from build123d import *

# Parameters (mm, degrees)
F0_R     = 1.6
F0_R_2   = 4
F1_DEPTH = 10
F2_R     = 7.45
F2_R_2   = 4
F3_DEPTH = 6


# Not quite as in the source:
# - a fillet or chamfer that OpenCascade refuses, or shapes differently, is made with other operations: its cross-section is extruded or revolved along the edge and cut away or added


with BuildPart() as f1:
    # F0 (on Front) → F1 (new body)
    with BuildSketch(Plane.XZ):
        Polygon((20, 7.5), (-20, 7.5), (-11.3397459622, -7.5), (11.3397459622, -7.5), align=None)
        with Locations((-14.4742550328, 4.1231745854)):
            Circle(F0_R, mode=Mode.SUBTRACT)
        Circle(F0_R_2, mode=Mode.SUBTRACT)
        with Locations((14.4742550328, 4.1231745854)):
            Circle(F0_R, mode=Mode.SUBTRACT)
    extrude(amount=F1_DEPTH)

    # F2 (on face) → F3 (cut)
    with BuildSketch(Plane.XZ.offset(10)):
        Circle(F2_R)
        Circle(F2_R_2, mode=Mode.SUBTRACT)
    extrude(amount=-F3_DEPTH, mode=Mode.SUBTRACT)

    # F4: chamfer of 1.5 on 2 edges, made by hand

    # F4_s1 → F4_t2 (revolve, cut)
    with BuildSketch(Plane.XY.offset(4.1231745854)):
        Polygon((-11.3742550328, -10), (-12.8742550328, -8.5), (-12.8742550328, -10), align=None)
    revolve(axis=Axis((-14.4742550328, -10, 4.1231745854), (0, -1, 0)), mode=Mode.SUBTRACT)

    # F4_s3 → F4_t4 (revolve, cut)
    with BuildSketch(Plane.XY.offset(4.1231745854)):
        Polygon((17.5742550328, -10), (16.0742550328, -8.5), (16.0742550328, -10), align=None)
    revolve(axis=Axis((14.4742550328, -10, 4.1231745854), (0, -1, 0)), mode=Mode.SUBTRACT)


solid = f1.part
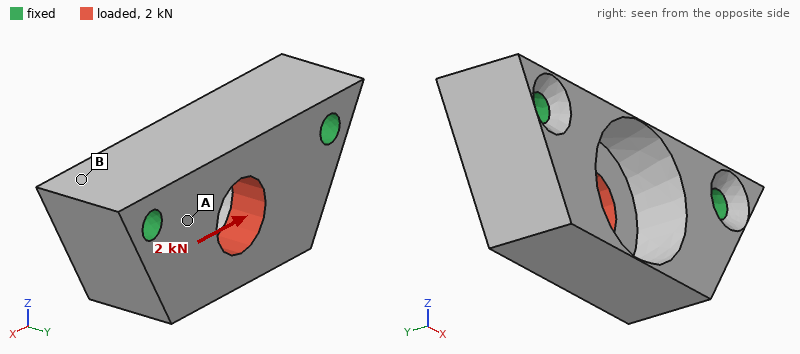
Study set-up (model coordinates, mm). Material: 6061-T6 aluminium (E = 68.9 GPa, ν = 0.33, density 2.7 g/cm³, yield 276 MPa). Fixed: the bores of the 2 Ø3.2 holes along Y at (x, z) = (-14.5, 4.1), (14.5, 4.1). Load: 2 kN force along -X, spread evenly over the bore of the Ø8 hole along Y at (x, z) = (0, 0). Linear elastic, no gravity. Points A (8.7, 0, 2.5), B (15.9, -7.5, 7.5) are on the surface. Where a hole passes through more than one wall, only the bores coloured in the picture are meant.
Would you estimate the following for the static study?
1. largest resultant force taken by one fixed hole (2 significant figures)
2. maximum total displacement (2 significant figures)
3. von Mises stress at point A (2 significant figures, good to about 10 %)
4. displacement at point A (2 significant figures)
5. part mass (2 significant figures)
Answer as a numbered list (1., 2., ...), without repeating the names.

1. 1.0 kN
2. 7.2 µm
3. 23 MPa
4. 2.2 µm
5. 8.8 g
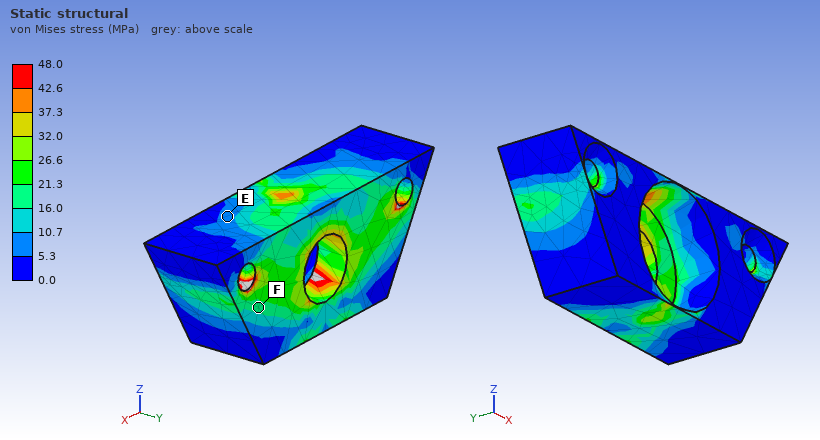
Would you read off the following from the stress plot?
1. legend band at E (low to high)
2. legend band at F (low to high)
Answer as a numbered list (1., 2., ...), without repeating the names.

1. 5.3 to 10.7 MPa
2. 16.0 to 21.3 MPa
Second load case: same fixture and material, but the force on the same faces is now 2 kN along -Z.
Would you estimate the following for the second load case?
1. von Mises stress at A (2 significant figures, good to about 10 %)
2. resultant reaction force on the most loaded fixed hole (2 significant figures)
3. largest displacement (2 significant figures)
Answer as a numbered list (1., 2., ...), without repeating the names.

1. 35 MPa
2. 1.1 kN
3. 16 µm
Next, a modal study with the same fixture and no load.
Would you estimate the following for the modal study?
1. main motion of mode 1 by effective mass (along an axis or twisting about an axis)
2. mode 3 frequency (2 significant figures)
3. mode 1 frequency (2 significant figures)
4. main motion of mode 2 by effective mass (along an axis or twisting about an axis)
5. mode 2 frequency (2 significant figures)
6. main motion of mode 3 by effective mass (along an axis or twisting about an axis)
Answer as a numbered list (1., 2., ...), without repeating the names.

1. along Y
2. 40 kHz
3. 28 kHz
4. along X
5. 35 kHz
6. along Z
